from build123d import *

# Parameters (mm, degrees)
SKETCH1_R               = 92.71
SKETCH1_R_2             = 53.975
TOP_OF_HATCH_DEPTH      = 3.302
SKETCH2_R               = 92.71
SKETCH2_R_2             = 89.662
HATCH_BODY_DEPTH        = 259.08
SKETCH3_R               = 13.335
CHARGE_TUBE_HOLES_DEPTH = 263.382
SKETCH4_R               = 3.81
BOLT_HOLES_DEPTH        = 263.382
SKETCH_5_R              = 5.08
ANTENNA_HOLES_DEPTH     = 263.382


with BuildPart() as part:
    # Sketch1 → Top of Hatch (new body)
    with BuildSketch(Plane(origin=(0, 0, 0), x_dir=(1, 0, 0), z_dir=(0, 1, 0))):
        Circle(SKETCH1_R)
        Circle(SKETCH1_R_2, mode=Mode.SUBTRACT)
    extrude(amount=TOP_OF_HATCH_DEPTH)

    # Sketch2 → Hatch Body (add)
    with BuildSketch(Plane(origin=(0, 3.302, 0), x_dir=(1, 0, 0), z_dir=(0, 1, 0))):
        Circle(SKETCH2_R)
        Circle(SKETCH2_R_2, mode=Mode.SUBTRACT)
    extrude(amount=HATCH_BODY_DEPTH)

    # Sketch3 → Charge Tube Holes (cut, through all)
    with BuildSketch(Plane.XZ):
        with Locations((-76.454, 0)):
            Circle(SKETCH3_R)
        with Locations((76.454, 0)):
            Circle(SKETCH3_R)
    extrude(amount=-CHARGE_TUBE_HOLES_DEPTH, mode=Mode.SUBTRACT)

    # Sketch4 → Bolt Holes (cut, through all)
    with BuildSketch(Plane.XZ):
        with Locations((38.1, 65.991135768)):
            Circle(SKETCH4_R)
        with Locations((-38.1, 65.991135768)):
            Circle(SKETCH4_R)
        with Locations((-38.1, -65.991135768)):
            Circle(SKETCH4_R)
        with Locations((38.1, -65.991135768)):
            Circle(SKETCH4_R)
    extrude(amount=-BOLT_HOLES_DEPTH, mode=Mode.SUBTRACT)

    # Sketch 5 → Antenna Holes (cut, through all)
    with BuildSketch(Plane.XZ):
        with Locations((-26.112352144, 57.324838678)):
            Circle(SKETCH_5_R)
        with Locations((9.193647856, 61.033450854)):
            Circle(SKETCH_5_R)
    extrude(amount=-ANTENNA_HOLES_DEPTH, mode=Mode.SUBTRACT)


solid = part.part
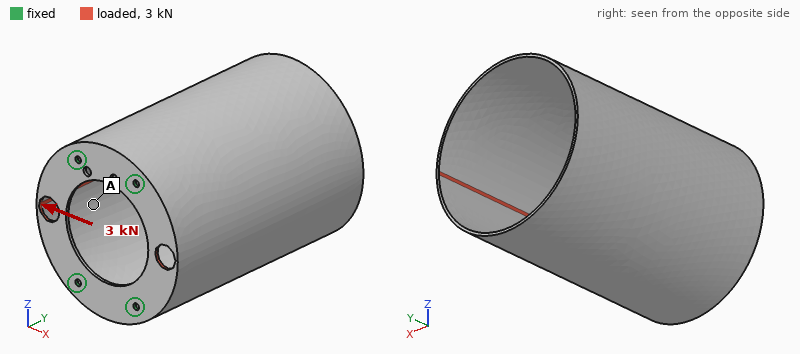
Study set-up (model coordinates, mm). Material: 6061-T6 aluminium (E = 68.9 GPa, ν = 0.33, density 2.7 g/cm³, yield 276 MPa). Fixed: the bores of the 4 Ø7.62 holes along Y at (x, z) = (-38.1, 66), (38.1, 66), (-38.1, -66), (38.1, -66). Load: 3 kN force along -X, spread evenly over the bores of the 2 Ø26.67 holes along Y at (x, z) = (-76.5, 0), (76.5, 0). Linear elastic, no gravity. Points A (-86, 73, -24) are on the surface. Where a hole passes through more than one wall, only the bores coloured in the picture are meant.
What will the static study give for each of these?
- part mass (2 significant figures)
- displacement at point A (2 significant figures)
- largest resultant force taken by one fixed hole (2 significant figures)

1.4 kg
0.35 mm
2.2 kN
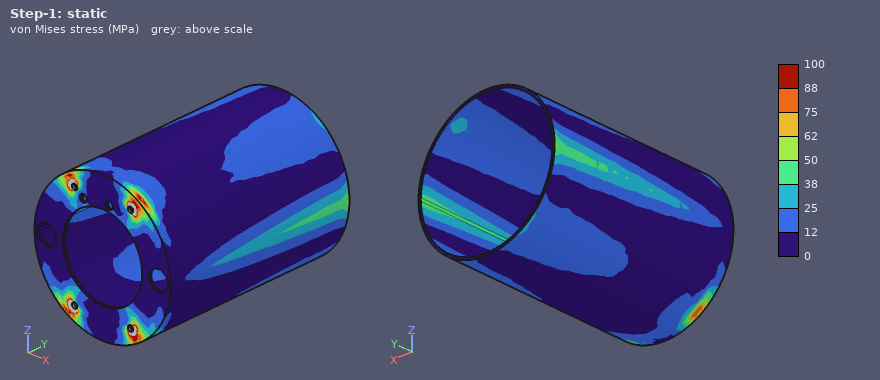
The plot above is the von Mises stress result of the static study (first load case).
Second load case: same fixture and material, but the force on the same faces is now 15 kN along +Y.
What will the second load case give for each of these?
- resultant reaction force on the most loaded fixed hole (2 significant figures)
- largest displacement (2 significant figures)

4.1 kN
2.5 mm
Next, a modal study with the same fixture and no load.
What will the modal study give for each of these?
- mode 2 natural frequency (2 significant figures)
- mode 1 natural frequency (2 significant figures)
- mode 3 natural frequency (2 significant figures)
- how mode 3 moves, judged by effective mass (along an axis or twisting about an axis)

300 Hz
260 Hz
310 Hz
along X
